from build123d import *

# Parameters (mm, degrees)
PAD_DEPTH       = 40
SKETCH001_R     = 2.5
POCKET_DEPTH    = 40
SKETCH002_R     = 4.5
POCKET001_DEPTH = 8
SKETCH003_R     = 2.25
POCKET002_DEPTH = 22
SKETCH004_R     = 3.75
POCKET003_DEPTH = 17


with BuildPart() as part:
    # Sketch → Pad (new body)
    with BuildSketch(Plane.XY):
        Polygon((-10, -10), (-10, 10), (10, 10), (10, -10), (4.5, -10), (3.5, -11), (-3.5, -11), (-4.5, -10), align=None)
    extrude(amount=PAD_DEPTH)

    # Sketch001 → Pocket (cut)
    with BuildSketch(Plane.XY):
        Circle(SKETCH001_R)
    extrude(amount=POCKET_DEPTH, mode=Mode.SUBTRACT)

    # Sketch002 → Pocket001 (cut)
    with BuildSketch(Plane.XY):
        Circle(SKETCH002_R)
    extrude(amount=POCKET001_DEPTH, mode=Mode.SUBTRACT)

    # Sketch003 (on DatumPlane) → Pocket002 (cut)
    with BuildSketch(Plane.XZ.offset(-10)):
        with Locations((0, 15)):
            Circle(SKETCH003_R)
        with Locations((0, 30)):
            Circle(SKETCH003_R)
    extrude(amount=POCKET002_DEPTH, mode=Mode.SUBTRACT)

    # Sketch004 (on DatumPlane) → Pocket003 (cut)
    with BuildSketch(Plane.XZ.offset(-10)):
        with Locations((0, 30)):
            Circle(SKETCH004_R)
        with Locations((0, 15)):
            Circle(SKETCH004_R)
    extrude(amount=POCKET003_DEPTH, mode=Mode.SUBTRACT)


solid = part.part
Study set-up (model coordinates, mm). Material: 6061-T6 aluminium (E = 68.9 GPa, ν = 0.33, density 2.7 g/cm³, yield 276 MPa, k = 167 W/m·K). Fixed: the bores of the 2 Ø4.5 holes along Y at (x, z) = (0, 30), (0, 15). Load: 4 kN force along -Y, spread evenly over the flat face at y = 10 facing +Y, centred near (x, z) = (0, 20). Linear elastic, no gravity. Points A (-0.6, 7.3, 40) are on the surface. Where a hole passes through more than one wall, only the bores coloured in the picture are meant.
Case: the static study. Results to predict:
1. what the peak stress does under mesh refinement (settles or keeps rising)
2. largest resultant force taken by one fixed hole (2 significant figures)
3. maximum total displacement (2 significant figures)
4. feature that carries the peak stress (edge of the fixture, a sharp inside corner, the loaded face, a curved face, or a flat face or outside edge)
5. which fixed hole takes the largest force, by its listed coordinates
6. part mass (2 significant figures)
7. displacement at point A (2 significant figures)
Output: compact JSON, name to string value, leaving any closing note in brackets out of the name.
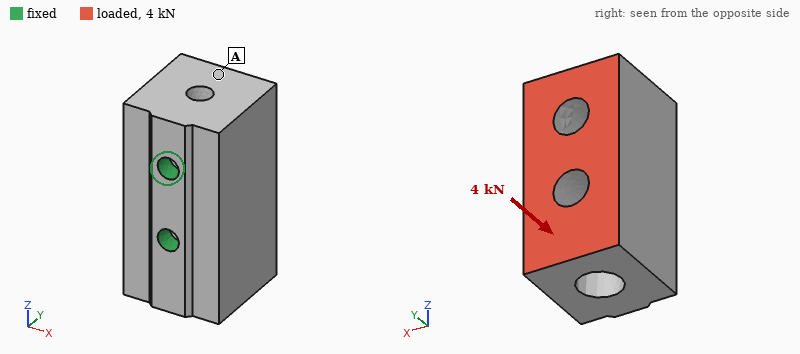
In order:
{"what the peak stress does under mesh refinement": "keeps rising", "largest resultant force taken by one fixed hole": "2.6 kN", "maximum total displacement": "15 µm", "feature that carries the peak stress": "edge of the fixture", "which fixed hole takes the largest force, by its listed coordinates": "(0, 15)", "part mass": "37 g", "displacement at point A": "4.0 µm"}
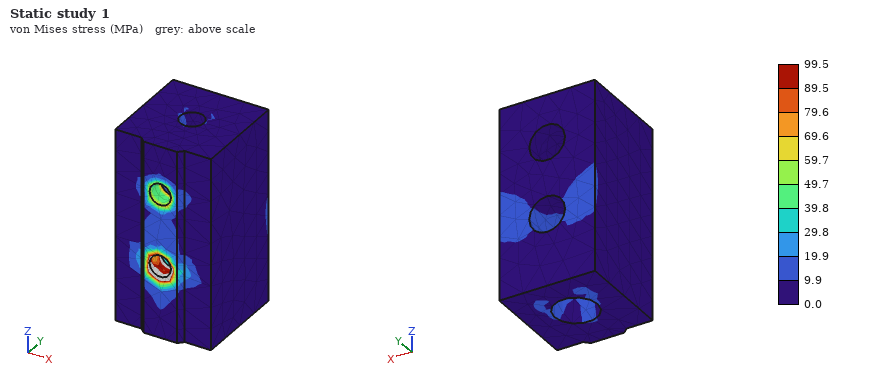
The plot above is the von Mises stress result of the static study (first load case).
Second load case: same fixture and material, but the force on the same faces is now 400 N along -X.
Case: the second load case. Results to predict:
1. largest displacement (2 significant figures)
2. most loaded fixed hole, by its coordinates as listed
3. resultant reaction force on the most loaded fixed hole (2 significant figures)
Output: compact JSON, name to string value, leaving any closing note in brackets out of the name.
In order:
{"largest displacement": "19 µm", "most loaded fixed hole, by its coordinates as listed": "(0, 15)", "resultant reaction force on the most loaded fixed hole": "260 N"}
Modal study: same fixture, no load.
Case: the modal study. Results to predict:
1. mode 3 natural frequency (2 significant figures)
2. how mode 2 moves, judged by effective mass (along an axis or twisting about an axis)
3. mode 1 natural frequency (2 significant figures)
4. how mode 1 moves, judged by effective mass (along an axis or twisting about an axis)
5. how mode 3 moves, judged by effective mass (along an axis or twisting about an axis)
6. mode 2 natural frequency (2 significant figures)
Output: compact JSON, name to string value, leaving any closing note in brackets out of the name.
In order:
{"mode 3 natural frequency": "15 kHz", "how mode 2 moves, judged by effective mass": "along Z", "mode 1 natural frequency": "6400 Hz", "how mode 1 moves, judged by effective mass": "along X", "how mode 3 moves, judged by effective mass": "twisting about Y", "mode 2 natural frequency": "12 kHz"}
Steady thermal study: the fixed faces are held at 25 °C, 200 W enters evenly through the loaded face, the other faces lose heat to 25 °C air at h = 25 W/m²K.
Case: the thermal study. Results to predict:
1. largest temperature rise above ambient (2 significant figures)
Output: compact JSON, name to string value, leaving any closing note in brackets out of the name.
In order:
{"largest temperature rise above ambient": "66 K"}
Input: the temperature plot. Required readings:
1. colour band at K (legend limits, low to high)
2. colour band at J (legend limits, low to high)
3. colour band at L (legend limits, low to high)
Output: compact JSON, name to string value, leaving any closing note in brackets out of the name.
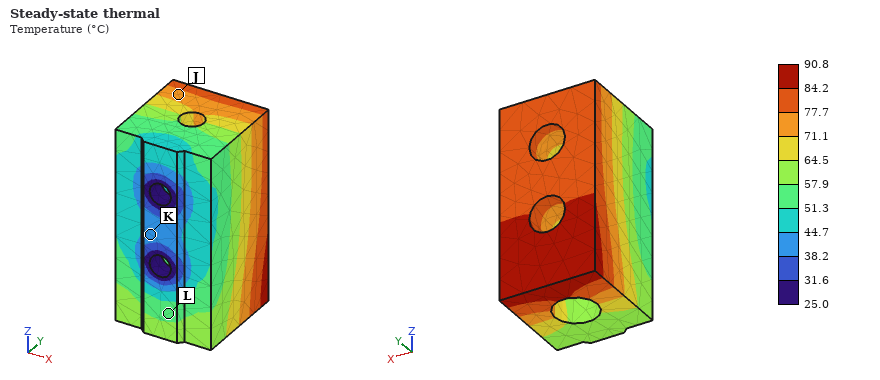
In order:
{"colour band at K": "38.2 to 44.7 °C", "colour band at J": "71.1 to 77.7 °C", "colour band at L": "51.3 to 57.9 °C"}
